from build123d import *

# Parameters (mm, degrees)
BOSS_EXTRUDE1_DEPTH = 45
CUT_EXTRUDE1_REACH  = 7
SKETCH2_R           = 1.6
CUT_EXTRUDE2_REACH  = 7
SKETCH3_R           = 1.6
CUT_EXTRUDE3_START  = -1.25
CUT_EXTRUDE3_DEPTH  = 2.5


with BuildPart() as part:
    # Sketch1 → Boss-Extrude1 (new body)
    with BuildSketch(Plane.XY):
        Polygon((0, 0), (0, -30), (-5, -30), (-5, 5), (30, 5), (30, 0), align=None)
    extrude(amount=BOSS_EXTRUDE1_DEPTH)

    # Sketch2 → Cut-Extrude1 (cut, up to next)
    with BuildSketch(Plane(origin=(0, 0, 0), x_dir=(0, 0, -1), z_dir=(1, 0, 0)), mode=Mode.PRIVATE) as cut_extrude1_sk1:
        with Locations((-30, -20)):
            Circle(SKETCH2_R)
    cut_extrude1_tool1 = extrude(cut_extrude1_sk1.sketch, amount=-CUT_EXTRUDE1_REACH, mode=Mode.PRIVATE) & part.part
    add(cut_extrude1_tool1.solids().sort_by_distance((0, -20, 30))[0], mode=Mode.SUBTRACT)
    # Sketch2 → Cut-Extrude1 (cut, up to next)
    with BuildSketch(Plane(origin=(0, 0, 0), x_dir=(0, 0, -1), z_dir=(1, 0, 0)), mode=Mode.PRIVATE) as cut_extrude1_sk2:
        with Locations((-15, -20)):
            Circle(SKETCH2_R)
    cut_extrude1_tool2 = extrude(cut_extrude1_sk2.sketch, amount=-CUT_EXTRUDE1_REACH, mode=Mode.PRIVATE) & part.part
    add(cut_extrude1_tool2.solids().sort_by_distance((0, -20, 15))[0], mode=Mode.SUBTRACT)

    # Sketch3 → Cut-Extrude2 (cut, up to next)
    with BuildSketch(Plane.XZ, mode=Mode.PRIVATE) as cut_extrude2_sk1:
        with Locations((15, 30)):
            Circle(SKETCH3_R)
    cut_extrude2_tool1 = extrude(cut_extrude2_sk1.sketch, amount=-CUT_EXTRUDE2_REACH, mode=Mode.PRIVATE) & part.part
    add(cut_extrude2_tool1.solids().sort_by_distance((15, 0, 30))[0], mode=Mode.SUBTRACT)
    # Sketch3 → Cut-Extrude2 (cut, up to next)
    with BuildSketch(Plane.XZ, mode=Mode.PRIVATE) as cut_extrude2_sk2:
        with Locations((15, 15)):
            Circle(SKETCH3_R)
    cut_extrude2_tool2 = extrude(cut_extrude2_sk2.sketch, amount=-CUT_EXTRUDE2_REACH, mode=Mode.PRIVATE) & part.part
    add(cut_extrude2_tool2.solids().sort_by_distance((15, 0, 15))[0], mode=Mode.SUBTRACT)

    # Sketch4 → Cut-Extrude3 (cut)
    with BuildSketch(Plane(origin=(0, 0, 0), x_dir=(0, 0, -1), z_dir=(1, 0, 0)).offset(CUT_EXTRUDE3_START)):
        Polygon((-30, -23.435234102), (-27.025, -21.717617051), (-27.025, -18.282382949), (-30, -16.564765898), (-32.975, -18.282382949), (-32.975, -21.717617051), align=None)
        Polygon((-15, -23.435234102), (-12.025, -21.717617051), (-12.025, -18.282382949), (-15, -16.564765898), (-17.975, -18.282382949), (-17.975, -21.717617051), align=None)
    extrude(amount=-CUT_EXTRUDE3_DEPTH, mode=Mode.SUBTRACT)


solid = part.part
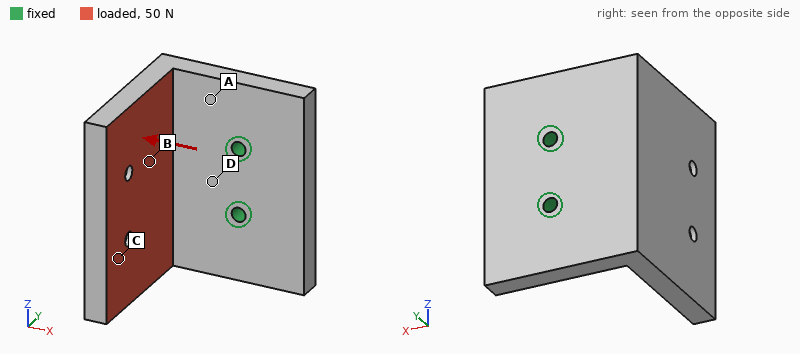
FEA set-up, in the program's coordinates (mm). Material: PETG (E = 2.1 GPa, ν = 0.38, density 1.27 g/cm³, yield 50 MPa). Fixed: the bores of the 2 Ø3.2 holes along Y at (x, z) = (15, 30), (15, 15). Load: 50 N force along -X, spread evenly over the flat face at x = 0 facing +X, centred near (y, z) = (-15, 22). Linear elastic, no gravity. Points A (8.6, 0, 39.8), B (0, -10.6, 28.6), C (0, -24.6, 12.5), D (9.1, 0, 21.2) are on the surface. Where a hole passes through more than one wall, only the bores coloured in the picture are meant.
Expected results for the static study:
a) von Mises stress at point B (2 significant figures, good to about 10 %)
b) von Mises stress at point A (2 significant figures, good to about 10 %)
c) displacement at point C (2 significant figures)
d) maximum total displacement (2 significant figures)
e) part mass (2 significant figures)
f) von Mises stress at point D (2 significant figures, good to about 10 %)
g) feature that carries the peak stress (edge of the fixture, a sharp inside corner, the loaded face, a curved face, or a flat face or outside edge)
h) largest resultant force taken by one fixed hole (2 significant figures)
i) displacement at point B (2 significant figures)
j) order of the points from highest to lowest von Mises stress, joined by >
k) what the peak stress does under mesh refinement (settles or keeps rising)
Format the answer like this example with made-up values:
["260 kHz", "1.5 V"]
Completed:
["1.5 MPa", "3.8 MPa", "0.57 mm", "0.73 mm", "18 g", "4.6 MPa", "edge of the fixture", "25 N", "0.27 mm", "D > A > B > C", "keeps rising"]
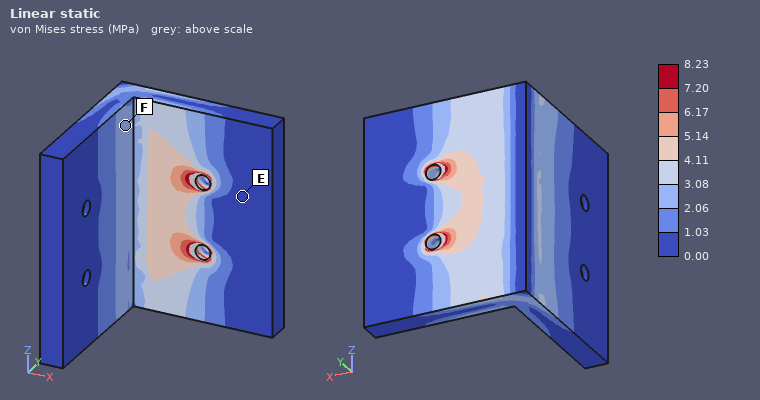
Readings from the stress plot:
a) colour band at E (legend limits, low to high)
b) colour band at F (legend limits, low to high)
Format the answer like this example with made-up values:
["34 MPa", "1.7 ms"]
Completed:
["0.00 to 1.03 MPa", "2.06 to 3.08 MPa"]
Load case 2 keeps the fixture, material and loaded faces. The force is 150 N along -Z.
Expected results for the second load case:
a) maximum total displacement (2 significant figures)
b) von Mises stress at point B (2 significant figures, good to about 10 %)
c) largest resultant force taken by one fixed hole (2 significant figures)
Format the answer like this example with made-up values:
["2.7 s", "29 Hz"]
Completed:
["0.80 mm", "3.7 MPa", "190 N"]
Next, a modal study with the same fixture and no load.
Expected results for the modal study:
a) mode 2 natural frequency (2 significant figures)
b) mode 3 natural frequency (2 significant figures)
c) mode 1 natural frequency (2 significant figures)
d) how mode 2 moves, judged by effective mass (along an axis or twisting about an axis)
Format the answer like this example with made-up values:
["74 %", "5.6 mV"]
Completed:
["840 Hz", "1600 Hz", "530 Hz", "along Z"]
